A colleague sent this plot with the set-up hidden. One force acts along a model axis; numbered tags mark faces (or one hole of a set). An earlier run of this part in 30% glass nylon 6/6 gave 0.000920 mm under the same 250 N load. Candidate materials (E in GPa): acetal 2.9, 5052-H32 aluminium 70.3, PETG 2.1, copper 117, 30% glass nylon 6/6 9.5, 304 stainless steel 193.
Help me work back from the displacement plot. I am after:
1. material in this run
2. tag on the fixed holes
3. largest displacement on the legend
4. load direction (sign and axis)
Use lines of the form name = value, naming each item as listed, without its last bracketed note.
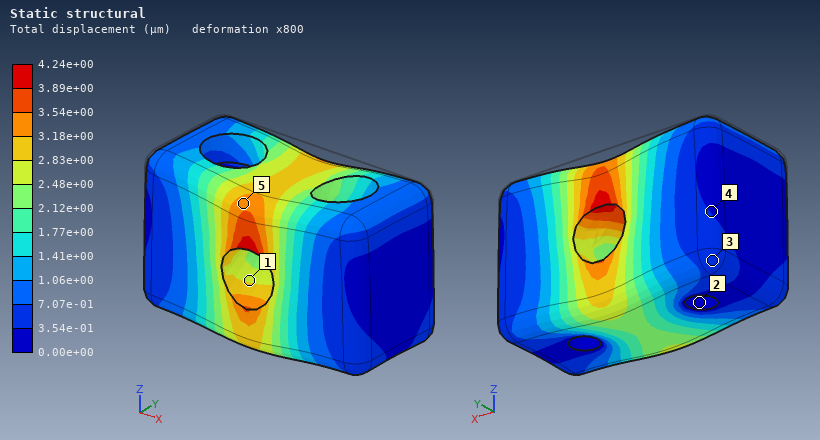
material in this run = PETG
tag on the fixed holes = 2
largest displacement on the legend = 4.24e+00 µm
load direction = -Z
